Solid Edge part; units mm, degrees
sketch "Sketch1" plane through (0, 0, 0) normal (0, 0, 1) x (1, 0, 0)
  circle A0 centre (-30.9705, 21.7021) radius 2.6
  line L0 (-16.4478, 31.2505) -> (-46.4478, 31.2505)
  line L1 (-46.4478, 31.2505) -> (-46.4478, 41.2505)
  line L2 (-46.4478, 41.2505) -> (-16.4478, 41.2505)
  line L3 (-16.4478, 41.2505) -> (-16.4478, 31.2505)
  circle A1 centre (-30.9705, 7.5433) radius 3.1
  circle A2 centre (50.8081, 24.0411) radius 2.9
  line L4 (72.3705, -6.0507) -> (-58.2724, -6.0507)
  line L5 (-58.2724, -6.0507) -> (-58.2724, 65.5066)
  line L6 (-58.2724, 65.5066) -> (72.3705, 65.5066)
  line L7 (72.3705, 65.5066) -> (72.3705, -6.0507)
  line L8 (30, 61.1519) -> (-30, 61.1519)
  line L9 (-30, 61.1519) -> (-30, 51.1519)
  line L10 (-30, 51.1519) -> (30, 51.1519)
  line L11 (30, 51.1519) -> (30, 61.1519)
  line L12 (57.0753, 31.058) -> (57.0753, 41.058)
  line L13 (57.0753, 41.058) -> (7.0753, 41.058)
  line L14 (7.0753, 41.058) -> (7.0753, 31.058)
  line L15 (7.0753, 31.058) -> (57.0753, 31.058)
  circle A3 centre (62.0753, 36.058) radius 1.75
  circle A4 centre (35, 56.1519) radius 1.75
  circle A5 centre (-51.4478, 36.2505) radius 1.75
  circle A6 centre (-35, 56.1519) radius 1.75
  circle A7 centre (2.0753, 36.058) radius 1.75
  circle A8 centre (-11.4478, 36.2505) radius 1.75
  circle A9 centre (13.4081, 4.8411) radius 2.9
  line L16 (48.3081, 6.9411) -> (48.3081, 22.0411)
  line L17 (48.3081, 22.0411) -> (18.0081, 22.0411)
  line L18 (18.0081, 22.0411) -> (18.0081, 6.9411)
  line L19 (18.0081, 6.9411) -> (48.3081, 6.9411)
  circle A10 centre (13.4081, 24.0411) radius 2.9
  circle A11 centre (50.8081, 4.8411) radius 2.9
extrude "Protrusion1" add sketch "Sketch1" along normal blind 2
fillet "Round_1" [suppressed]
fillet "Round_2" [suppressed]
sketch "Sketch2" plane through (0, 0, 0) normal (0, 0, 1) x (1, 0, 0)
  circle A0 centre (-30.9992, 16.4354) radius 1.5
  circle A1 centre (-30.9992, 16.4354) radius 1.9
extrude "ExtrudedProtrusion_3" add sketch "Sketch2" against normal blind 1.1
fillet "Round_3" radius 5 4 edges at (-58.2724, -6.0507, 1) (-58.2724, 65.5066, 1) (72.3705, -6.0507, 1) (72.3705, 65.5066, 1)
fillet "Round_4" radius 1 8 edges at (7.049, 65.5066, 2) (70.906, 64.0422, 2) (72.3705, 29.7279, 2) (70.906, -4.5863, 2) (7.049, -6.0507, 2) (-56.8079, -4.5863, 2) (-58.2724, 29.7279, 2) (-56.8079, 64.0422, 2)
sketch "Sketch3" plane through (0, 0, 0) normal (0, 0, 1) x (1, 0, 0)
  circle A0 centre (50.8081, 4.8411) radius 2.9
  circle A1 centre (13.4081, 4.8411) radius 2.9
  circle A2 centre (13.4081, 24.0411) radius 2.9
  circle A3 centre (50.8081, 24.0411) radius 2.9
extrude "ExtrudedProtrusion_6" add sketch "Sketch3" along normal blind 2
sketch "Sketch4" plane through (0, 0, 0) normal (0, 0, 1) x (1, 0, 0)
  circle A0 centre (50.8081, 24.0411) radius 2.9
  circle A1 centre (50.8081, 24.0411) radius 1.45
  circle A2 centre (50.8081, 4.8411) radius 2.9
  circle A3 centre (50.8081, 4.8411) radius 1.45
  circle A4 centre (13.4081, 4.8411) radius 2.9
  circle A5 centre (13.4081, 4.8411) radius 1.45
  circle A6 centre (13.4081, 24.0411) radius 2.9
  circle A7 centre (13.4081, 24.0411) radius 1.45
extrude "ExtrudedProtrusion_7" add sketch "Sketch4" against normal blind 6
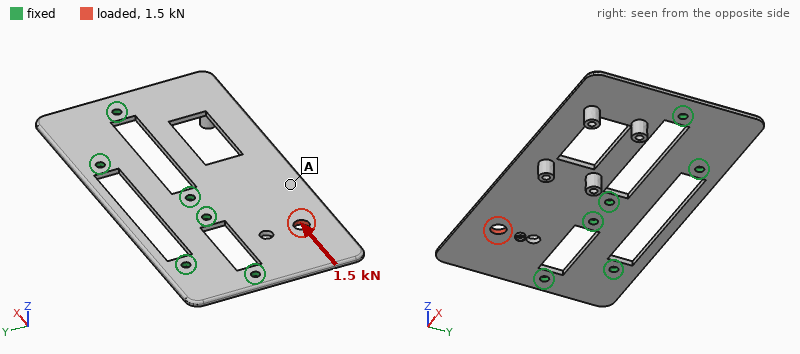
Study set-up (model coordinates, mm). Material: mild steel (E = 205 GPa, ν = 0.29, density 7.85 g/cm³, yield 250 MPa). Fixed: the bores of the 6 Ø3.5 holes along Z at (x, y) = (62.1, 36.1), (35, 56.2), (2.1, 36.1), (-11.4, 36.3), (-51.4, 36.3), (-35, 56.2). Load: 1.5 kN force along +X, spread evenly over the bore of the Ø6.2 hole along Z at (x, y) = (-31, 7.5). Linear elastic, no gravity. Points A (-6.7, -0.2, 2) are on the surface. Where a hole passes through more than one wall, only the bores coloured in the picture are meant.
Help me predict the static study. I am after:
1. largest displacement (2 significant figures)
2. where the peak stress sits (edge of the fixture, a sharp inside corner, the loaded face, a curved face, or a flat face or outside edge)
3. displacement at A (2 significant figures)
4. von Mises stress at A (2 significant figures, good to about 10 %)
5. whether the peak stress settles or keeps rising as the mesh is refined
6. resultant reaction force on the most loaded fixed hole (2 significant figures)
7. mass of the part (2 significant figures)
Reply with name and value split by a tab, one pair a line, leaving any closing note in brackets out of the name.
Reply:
largest displacement	8.9 µm
where the peak stress sits	edge of the fixture
displacement at A	6.8 µm
von Mises stress at A	8.1 MPa
whether the peak stress settles or keeps rising as the mesh is refined	keeps rising
resultant reaction force on the most loaded fixed hole	730 N
mass of the part	120 g
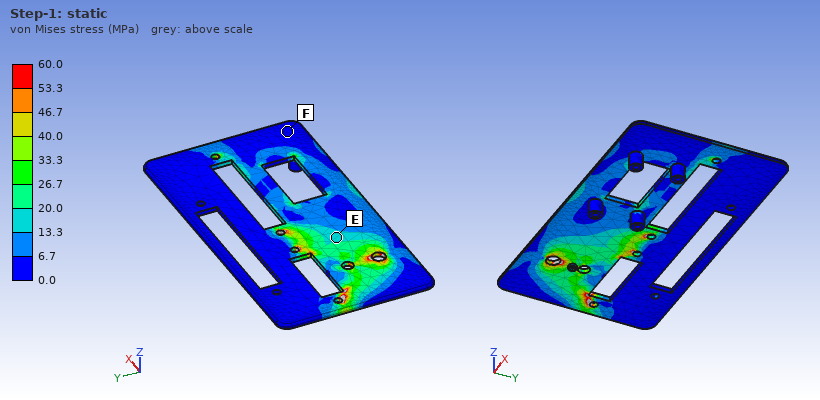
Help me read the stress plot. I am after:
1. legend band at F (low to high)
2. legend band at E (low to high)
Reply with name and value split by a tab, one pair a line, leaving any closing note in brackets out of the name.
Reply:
legend band at F	0.0 to 6.7 MPa
legend band at E	13.3 to 20.0 MPa
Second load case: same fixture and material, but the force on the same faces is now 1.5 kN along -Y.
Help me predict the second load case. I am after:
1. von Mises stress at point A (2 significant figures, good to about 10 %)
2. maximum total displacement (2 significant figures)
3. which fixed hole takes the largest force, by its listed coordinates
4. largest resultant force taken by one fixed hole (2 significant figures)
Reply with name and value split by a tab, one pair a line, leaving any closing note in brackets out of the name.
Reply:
von Mises stress at point A	3.6 MPa
maximum total displacement	6.3 µm
which fixed hole takes the largest force, by its listed coordinates	(-51.4, 36.3)
largest resultant force taken by one fixed hole	770 N
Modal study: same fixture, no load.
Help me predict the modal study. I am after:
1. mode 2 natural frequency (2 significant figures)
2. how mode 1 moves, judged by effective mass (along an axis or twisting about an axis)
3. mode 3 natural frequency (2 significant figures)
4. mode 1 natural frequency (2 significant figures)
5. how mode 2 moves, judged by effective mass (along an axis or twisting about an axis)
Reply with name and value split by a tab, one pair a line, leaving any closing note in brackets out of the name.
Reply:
mode 2 natural frequency	980 Hz
how mode 1 moves, judged by effective mass	along Z
mode 3 natural frequency	1600 Hz
mode 1 natural frequency	670 Hz
how mode 2 moves, judged by effective mass	twisting about Y
